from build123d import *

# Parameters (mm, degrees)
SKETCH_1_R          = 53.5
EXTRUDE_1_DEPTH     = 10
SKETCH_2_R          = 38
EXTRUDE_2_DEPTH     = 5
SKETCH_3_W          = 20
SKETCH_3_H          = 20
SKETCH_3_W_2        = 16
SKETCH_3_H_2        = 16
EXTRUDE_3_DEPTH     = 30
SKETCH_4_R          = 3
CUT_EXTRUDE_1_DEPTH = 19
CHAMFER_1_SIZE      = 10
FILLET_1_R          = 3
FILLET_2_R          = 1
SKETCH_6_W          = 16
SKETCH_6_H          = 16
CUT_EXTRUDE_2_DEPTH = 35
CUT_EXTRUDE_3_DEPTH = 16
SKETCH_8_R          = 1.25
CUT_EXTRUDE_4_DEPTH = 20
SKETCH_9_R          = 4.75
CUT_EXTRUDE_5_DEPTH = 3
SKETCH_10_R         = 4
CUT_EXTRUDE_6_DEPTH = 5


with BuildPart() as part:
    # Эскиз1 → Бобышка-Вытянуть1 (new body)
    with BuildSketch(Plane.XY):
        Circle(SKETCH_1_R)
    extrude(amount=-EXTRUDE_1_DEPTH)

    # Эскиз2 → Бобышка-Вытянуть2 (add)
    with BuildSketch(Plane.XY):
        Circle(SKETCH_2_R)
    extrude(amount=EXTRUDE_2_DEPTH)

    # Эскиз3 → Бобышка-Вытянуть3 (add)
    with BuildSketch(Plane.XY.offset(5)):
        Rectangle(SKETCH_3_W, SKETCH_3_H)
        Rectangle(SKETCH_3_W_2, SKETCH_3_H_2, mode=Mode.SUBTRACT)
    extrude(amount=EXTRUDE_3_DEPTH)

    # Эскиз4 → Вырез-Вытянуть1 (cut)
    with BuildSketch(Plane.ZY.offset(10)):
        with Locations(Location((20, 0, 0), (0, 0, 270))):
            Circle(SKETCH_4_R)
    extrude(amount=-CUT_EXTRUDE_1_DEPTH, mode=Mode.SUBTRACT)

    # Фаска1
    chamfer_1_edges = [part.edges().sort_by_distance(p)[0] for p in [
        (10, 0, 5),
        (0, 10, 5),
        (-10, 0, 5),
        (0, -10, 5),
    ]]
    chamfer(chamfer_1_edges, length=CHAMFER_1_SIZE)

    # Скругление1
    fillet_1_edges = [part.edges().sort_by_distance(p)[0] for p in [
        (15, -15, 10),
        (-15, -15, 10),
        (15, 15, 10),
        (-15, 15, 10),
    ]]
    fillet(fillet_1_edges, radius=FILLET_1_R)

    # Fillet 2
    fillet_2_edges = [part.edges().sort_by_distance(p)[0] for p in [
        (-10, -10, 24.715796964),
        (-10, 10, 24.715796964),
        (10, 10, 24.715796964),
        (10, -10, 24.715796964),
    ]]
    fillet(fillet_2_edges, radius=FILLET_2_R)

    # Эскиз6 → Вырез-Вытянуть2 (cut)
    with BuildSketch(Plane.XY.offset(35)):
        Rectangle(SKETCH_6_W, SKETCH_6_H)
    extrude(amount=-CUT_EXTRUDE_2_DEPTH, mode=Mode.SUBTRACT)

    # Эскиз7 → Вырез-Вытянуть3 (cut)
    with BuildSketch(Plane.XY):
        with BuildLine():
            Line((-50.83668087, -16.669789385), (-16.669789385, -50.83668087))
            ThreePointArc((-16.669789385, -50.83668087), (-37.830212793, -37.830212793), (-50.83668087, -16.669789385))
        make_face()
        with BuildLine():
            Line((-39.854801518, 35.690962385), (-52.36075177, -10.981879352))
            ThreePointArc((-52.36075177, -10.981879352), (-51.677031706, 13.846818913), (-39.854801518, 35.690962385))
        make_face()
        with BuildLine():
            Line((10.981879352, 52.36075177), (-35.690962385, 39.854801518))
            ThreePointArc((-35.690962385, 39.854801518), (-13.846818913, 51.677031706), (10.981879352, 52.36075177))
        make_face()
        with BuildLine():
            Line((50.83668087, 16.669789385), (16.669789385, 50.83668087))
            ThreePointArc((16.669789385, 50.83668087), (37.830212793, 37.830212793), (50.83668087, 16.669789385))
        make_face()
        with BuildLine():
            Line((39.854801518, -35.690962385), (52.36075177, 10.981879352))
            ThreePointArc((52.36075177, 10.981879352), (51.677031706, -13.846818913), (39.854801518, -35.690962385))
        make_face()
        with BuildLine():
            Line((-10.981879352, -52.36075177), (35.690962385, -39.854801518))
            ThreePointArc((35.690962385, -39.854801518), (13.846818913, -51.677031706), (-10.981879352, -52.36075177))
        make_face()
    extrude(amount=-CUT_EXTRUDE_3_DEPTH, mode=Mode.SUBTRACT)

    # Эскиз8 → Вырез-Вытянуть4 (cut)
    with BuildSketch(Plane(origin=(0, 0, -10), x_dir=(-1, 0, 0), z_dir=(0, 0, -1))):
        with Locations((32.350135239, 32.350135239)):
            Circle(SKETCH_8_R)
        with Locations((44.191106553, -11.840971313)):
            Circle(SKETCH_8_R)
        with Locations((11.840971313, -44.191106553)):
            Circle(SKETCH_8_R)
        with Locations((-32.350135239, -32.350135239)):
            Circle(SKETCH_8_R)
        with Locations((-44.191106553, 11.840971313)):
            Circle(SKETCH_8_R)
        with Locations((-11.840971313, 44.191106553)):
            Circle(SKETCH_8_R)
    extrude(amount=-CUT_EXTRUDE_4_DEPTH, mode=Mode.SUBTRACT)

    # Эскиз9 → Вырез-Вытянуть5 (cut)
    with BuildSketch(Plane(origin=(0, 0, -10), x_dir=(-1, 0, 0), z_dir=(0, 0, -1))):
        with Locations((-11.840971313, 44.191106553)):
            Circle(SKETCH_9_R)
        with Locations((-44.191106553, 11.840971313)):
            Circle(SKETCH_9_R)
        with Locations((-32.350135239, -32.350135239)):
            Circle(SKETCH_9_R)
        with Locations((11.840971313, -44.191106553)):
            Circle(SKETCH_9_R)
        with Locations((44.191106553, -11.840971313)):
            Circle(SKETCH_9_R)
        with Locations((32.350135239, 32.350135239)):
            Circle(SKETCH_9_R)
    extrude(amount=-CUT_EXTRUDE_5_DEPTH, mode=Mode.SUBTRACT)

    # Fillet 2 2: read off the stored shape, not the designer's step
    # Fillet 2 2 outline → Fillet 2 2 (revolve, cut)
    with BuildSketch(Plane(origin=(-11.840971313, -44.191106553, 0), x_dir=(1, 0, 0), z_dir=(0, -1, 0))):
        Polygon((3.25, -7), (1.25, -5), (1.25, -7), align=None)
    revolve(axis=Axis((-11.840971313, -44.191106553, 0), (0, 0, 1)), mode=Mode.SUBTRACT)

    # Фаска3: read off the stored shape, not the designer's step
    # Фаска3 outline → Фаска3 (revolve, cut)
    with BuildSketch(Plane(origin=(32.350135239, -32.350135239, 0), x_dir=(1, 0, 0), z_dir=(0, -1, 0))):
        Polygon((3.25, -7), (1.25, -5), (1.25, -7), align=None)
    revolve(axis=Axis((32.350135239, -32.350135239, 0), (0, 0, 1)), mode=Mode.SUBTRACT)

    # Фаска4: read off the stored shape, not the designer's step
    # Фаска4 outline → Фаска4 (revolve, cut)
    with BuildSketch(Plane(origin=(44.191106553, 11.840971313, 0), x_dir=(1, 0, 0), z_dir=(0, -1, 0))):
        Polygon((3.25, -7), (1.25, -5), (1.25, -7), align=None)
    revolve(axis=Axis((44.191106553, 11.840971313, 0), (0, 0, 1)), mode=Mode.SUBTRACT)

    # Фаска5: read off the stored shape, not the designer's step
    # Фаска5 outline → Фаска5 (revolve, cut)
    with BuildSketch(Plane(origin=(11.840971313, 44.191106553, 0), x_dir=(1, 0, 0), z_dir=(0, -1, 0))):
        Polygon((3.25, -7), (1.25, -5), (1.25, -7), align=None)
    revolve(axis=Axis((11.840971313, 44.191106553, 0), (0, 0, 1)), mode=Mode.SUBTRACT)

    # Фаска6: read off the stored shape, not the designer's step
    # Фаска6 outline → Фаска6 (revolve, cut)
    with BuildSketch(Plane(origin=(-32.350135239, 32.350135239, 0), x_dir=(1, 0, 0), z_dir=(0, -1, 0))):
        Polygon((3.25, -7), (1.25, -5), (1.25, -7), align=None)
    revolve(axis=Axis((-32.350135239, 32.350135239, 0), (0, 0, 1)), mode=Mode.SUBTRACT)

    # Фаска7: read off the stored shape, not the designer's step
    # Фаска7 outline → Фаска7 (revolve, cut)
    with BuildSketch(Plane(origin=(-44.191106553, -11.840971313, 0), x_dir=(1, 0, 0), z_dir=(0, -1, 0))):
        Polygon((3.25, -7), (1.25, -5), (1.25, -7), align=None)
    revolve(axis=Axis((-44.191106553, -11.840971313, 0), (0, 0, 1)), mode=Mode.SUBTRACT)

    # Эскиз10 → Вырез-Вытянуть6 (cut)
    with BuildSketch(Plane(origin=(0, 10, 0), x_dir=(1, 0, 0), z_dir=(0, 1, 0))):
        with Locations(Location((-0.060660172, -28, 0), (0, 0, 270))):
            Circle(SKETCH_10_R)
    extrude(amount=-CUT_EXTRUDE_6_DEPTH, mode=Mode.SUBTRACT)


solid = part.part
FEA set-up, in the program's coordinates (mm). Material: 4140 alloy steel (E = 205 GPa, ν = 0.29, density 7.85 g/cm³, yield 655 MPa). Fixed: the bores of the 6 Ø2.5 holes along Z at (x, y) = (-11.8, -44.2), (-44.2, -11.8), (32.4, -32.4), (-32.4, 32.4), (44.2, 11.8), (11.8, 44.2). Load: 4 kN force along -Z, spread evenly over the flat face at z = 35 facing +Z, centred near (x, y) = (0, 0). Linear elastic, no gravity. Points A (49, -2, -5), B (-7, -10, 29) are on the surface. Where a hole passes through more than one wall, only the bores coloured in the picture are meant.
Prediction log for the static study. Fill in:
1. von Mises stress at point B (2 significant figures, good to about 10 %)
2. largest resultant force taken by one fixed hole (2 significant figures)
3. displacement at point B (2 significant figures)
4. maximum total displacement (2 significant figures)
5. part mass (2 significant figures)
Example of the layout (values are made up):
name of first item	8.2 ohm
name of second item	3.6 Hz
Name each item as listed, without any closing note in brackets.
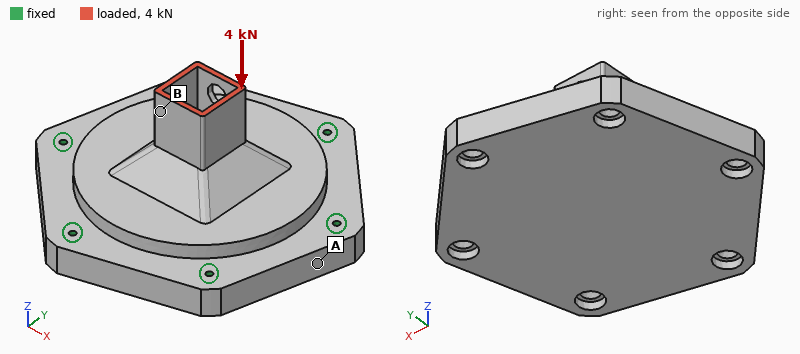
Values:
von Mises stress at point B	29 MPa
largest resultant force taken by one fixed hole	670 N
displacement at point B	7.0 µm
maximum total displacement	11 µm
part mass	850 g
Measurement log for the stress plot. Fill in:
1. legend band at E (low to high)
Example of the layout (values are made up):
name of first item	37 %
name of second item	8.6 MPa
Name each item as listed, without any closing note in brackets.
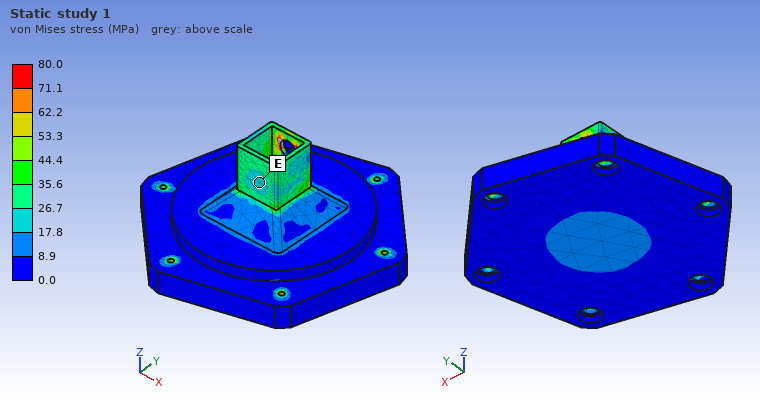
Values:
legend band at E	17.8 to 26.7 MPa
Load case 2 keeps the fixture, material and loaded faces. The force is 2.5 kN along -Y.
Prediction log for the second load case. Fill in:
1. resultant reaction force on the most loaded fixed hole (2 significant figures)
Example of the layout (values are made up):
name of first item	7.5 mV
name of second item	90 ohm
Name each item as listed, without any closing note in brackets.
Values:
resultant reaction force on the most loaded fixed hole	830 N
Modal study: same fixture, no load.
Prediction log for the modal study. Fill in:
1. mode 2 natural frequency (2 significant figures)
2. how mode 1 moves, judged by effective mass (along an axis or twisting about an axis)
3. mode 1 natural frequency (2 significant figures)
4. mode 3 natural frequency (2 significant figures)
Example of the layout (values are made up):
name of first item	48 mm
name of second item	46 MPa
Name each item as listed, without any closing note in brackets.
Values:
mode 2 natural frequency	12 kHz
how mode 1 moves, judged by effective mass	along Z
mode 1 natural frequency	7200 Hz
mode 3 natural frequency	12 kHz
